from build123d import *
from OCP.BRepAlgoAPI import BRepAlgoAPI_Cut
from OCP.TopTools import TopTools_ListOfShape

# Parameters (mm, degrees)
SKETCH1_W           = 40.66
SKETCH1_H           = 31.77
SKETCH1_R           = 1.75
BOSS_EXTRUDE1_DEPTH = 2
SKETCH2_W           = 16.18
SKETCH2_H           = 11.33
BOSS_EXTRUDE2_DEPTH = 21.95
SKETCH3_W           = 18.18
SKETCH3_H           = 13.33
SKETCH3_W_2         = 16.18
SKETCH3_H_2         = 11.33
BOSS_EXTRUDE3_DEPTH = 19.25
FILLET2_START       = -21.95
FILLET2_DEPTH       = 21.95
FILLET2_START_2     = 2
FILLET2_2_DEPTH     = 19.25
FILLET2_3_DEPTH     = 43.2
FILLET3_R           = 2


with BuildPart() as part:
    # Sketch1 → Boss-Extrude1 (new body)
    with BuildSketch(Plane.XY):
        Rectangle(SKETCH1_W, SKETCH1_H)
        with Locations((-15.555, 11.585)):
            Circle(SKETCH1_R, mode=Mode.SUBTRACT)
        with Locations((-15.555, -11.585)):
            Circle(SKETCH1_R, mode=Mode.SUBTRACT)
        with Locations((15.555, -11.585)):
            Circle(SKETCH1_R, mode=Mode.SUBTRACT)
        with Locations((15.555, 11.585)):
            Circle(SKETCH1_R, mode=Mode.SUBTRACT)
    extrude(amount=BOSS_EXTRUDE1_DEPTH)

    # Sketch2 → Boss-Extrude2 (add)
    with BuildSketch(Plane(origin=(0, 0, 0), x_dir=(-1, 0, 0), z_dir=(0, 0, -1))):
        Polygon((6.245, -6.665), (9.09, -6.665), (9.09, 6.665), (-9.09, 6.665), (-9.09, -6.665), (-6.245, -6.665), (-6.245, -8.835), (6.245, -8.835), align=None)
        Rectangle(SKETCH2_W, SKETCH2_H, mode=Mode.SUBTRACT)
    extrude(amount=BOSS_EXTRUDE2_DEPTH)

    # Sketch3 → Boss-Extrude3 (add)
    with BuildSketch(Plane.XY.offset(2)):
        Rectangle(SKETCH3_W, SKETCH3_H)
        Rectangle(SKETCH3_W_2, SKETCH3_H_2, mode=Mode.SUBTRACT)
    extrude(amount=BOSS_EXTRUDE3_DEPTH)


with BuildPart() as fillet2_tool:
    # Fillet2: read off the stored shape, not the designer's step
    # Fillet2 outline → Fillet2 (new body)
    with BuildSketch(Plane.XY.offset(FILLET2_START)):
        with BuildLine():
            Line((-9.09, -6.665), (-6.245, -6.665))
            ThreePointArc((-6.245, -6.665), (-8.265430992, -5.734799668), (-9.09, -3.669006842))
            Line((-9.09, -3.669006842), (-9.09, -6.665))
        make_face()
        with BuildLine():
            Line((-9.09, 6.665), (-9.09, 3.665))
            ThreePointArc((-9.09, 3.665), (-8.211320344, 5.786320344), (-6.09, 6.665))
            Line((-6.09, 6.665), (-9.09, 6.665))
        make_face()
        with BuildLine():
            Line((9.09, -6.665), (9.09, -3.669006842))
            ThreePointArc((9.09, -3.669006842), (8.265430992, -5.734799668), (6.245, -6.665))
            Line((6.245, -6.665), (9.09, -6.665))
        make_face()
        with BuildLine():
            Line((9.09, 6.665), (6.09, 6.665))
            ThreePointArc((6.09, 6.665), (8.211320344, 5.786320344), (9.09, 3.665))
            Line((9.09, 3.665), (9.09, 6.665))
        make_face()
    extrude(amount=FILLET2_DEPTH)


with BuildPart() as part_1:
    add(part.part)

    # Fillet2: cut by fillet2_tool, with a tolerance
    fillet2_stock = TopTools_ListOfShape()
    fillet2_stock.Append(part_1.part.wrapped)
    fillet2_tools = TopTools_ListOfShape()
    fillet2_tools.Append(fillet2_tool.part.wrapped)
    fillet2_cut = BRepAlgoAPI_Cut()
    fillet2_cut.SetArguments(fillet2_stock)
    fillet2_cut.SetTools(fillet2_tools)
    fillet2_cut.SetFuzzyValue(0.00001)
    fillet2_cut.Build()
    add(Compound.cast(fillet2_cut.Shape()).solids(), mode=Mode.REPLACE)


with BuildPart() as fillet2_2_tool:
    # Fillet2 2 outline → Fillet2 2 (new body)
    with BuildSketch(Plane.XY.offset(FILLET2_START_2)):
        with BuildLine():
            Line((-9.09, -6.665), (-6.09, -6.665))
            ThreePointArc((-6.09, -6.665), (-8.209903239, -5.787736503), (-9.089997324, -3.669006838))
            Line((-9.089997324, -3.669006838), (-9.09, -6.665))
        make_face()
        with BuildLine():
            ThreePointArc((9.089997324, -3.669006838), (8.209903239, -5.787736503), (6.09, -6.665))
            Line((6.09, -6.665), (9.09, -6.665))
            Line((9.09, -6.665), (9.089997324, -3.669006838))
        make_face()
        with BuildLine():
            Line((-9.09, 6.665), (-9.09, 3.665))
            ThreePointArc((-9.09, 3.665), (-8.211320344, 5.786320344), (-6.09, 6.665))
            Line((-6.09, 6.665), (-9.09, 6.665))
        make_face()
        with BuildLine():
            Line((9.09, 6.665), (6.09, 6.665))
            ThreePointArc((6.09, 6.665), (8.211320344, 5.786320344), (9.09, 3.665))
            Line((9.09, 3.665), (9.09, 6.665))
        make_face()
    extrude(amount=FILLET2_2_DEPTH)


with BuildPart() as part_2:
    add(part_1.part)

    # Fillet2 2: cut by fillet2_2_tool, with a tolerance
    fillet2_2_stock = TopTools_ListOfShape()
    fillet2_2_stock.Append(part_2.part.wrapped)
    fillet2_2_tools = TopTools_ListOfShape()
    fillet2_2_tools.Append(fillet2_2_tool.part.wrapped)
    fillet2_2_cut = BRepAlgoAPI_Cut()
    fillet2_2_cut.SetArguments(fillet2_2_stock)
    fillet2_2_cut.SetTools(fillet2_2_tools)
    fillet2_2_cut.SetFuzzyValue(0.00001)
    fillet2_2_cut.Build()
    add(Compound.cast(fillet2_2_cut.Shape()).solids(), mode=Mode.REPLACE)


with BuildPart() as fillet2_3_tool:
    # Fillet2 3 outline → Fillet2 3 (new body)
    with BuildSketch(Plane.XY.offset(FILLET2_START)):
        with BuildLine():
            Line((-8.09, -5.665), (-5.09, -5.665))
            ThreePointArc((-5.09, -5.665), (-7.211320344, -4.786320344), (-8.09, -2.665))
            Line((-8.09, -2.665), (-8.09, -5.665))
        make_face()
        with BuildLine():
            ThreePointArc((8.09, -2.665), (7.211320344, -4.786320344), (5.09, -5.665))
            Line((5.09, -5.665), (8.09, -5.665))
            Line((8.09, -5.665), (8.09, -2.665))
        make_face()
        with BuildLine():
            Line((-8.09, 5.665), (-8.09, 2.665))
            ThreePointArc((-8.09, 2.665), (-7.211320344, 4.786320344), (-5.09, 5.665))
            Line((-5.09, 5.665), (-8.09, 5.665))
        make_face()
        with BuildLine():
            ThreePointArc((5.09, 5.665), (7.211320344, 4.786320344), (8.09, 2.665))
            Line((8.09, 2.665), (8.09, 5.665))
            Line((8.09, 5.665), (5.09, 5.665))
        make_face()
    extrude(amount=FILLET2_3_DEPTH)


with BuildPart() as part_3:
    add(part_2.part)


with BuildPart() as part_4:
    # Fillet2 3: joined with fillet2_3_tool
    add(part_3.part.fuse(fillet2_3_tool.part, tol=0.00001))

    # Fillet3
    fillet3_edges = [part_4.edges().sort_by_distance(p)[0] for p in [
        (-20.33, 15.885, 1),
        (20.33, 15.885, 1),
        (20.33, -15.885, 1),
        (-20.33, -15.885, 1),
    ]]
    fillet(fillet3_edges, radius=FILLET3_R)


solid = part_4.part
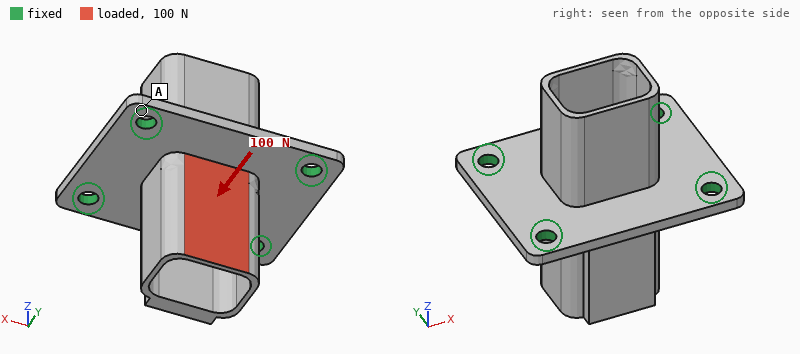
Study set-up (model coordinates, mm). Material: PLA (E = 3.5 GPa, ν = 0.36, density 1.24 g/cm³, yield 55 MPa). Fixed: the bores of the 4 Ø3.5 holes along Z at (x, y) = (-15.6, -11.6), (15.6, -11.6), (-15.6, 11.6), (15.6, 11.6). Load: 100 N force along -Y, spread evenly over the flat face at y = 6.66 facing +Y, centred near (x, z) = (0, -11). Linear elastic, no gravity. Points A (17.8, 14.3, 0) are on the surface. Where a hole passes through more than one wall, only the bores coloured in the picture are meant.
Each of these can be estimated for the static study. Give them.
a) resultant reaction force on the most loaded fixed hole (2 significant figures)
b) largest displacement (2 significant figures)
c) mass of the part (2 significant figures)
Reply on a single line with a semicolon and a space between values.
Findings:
42 N; 0.65 mm; 6.9 g
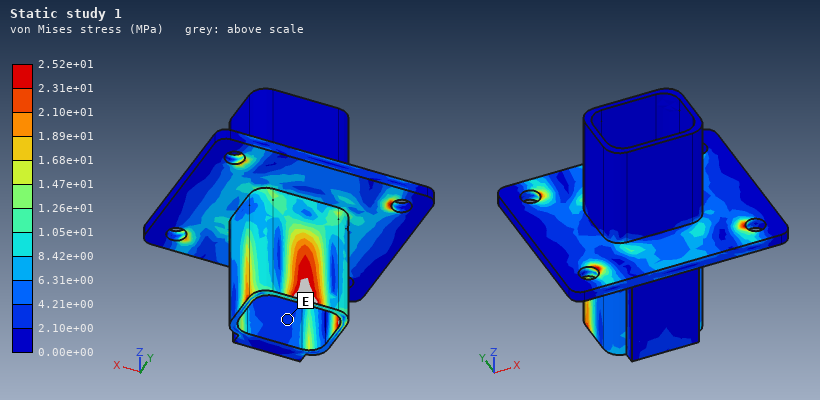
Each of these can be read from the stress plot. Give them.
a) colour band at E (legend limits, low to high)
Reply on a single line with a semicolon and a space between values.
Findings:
2.10e+00 to 4.21e+00 MPa
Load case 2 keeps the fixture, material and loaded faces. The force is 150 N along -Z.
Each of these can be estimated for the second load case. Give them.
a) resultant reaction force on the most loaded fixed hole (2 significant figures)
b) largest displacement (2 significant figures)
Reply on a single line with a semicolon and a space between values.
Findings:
63 N; 0.38 mm
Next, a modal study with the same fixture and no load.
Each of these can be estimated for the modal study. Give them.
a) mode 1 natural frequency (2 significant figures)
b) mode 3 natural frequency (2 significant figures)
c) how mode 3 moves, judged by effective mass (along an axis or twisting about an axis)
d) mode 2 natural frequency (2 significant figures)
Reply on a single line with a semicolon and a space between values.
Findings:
1800 Hz; 2500 Hz; along Z; 2300 Hz
